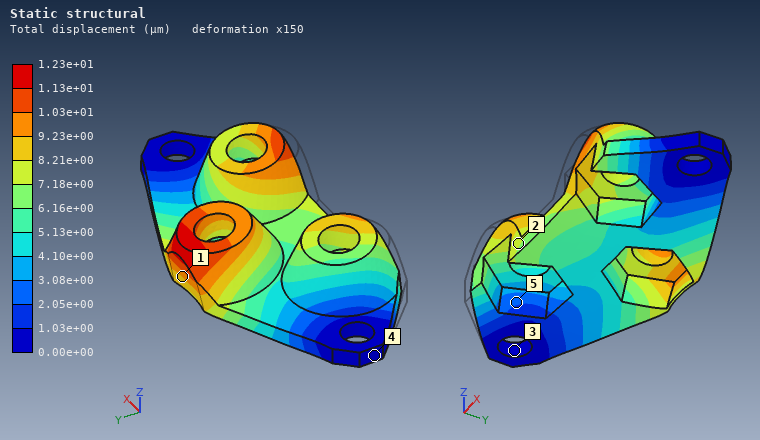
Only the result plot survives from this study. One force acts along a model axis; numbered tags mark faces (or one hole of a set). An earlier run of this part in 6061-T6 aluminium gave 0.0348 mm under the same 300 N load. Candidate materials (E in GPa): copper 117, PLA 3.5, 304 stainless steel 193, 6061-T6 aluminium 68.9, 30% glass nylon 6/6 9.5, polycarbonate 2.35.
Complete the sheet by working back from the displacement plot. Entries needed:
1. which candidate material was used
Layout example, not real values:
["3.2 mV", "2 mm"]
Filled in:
["304 stainless steel"]
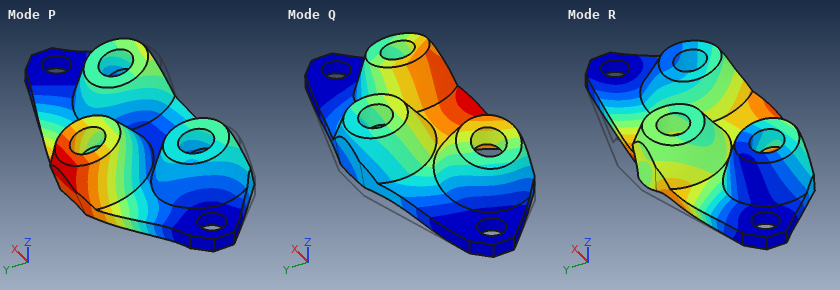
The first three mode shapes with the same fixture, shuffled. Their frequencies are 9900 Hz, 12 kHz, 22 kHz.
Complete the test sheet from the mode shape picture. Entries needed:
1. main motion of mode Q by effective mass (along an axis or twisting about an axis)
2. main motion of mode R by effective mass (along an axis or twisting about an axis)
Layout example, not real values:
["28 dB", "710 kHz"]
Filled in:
["along Z", "along Y"]
